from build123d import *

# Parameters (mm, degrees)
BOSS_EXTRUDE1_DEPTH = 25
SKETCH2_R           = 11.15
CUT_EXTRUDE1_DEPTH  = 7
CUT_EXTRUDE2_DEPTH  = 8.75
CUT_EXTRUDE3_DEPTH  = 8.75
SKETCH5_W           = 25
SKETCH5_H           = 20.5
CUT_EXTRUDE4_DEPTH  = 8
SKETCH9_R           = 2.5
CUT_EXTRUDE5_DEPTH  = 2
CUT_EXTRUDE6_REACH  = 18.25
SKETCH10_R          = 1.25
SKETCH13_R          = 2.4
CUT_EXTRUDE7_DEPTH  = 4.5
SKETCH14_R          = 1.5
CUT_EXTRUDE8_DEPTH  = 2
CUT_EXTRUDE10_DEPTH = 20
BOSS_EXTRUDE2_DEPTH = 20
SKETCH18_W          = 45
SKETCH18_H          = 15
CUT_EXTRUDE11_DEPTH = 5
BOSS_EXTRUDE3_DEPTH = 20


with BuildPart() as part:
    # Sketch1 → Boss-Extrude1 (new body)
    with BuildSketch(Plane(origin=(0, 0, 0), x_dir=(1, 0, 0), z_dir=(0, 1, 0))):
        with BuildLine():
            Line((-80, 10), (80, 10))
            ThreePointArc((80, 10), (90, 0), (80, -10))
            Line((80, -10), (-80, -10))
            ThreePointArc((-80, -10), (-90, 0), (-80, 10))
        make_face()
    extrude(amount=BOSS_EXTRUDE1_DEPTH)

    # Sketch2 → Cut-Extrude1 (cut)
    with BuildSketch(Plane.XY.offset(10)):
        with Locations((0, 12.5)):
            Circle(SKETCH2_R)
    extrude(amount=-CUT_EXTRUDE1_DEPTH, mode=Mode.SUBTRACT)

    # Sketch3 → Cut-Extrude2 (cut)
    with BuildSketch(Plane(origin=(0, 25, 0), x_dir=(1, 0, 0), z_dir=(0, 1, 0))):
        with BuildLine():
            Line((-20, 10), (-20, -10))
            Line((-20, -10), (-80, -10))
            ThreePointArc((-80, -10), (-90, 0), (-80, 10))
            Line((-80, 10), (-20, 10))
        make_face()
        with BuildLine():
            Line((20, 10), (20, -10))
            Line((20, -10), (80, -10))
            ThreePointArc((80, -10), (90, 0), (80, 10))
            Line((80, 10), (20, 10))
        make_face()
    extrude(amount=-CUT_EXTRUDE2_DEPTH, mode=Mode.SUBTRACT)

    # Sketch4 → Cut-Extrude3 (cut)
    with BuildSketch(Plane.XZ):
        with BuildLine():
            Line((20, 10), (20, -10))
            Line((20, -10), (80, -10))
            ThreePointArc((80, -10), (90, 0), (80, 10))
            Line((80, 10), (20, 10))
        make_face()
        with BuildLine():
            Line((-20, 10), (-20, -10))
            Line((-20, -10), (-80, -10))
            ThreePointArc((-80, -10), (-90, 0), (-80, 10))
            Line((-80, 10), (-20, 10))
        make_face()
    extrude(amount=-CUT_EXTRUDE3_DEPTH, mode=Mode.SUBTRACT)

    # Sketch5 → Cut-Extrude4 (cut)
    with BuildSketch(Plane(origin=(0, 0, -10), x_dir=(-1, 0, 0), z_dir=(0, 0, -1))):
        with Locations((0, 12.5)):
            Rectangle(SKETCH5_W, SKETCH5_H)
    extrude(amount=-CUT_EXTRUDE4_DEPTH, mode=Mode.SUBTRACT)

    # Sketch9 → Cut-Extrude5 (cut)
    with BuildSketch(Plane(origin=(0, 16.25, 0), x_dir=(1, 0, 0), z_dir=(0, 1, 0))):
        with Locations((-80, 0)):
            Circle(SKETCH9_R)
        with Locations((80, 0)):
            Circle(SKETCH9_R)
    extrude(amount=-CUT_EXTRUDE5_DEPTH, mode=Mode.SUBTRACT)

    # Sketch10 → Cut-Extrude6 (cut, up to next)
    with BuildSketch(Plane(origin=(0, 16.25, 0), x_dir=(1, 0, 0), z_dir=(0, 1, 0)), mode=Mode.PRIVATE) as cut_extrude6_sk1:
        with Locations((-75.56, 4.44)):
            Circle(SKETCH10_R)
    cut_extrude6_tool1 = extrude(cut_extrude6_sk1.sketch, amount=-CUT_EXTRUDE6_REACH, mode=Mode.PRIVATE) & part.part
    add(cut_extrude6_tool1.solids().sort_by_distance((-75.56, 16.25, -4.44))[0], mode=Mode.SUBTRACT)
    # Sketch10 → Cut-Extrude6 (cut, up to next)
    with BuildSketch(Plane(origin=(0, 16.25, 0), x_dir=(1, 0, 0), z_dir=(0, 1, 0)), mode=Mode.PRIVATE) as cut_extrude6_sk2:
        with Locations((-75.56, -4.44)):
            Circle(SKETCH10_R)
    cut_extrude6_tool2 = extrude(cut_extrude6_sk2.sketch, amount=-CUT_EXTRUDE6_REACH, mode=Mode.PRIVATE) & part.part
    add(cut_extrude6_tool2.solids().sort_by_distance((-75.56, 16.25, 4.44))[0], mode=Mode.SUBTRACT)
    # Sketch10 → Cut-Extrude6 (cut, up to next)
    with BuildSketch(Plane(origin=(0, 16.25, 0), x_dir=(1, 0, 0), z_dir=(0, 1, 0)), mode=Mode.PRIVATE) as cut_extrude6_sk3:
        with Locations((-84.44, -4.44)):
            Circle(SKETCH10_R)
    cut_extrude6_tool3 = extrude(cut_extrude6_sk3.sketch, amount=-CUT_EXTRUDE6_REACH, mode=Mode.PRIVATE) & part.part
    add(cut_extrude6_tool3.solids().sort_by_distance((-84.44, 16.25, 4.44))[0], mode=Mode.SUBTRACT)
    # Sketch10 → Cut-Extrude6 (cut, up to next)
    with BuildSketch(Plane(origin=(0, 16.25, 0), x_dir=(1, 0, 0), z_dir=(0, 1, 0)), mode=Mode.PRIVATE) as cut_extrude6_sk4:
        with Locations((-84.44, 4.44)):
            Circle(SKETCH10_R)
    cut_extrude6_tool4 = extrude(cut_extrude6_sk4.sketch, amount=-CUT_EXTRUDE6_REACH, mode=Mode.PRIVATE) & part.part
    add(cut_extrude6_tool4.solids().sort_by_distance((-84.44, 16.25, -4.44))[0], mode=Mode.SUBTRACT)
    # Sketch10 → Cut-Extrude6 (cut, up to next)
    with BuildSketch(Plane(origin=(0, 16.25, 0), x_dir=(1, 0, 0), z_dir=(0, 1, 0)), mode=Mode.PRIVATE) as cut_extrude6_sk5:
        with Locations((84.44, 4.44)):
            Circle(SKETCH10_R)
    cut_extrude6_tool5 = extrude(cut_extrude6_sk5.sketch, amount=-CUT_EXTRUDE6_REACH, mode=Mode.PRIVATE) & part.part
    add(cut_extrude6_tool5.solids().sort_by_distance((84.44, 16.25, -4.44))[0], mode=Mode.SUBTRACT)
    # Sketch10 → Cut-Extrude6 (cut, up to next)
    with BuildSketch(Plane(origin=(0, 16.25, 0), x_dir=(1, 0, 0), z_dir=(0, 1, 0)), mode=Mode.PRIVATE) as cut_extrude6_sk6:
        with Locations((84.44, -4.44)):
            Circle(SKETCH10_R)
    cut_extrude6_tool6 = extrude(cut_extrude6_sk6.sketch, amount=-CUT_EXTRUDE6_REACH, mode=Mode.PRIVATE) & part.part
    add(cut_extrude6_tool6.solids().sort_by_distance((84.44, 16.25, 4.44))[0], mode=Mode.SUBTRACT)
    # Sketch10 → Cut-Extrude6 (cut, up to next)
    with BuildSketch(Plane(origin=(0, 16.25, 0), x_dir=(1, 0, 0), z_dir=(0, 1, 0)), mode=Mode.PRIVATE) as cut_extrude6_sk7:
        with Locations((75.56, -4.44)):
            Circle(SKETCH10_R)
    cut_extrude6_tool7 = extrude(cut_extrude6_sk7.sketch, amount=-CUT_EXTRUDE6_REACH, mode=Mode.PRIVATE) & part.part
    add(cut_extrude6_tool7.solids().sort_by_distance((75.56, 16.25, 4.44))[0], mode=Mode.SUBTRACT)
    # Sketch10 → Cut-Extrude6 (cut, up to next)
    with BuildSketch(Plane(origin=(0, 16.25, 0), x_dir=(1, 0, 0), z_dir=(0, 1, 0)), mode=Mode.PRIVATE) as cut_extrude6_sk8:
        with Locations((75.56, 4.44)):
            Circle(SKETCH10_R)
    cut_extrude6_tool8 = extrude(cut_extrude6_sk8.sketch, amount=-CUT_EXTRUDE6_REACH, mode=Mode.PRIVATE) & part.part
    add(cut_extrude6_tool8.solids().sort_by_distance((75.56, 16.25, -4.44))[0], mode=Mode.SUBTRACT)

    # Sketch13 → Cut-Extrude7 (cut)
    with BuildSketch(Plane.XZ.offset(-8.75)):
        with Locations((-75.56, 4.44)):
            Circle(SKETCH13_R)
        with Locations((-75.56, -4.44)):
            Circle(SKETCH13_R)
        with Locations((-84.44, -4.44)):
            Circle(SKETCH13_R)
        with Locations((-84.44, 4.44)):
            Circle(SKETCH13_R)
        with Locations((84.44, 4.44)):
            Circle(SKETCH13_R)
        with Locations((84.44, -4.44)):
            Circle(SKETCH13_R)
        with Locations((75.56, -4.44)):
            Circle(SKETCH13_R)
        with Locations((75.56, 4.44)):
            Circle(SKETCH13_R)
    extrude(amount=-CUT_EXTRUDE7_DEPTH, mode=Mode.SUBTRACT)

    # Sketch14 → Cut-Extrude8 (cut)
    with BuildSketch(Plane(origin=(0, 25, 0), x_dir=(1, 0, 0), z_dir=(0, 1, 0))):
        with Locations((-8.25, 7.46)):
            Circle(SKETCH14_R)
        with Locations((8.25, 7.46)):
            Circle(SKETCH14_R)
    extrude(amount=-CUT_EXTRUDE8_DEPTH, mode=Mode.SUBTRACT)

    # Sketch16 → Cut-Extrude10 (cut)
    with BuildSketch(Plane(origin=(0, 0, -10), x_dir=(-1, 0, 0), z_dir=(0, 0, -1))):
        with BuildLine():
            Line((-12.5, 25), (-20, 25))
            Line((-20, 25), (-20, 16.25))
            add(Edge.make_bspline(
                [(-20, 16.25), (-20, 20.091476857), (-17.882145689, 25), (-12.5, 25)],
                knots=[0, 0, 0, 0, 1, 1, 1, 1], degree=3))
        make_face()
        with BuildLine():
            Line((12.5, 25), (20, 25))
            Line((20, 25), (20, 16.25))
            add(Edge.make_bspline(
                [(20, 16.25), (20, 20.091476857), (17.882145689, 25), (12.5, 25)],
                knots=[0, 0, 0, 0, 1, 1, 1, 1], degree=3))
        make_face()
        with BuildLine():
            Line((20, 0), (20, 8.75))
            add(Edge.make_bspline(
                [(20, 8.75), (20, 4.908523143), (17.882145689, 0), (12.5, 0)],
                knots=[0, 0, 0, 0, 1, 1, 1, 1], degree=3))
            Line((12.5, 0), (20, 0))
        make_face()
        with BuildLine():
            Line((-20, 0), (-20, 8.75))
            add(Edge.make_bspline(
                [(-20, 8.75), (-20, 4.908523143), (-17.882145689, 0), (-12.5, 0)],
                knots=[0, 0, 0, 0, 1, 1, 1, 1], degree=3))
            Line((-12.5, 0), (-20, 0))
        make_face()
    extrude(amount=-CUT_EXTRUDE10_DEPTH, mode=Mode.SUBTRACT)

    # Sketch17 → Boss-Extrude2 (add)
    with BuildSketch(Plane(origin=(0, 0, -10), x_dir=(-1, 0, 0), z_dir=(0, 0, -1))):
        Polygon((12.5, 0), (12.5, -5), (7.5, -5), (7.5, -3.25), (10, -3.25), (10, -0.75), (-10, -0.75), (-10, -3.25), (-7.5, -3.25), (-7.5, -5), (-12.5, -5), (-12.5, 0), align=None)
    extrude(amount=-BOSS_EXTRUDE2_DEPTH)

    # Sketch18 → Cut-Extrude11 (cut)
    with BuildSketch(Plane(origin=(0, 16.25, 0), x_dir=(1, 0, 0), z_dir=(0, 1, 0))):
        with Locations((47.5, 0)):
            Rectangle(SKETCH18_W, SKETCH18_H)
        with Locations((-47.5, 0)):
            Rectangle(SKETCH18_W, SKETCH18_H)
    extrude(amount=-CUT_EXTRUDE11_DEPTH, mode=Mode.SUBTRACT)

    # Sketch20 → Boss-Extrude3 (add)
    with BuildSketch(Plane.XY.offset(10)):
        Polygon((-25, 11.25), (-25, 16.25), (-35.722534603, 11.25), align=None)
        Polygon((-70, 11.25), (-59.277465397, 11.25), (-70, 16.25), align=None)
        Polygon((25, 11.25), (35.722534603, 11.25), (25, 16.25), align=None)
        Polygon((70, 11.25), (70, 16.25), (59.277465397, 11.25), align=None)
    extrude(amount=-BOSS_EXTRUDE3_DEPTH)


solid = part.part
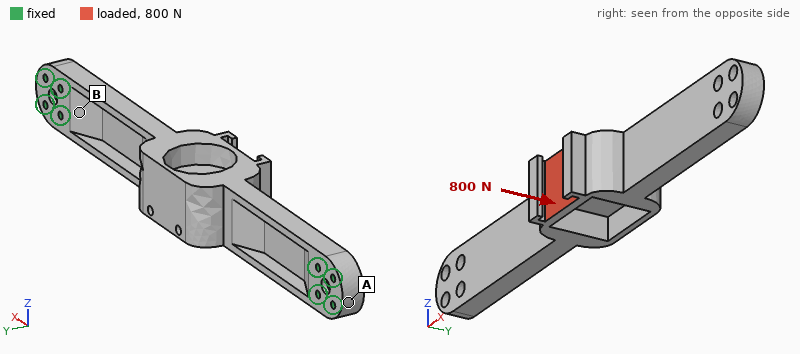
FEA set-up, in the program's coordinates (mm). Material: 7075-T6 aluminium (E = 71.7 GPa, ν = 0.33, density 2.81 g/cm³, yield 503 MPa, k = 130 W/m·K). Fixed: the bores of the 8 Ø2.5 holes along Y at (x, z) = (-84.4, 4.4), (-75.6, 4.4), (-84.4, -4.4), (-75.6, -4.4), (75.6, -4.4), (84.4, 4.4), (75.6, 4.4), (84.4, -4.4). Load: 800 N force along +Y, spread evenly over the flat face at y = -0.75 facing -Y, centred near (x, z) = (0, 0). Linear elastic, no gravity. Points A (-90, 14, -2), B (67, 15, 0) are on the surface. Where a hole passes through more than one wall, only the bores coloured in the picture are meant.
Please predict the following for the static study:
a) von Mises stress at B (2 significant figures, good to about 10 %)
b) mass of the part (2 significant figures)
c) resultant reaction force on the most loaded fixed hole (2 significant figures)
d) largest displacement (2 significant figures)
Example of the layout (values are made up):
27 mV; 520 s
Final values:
37 MPa; 77 g; 740 N; 0.24 mm
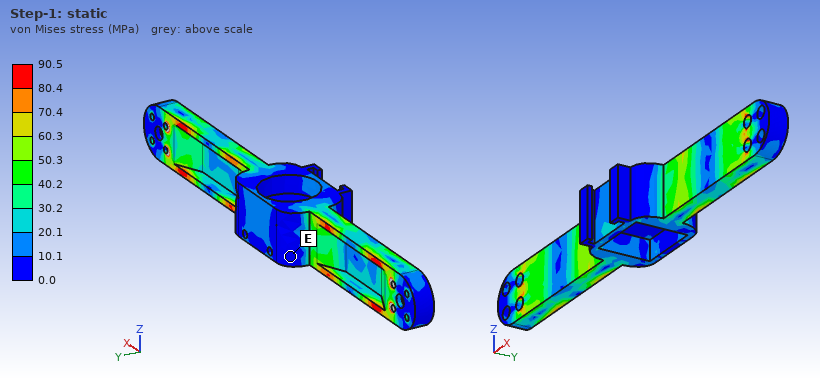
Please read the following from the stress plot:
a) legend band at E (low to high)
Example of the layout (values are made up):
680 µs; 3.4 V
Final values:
0.0 to 10.1 MPa
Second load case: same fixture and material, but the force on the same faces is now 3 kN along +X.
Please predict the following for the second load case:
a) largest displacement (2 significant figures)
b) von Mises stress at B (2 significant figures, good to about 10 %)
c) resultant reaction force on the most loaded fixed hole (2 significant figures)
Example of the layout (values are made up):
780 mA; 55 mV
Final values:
98 µm; 28 MPa; 790 N
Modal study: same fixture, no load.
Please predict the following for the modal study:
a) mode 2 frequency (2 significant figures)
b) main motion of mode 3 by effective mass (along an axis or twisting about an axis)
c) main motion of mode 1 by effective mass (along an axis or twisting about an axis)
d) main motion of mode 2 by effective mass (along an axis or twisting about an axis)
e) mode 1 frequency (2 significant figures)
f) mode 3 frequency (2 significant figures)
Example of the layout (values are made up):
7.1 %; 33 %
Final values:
1600 Hz; along Z; along Y; along Z; 1300 Hz; 2600 Hz
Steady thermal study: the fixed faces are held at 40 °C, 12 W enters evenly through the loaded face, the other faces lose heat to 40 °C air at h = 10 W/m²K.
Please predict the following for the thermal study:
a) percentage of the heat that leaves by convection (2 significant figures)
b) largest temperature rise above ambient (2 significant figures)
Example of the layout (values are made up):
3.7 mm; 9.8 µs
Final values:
19 %; 30 K
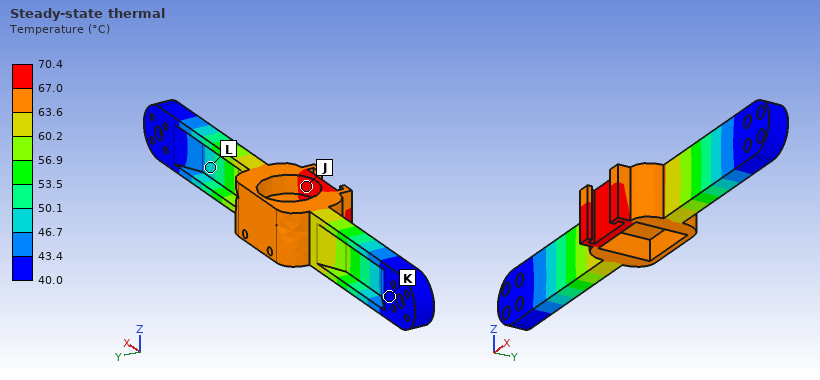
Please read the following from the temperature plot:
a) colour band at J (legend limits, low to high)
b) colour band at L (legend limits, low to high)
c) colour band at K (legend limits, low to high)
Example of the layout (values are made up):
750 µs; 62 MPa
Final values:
67.0 to 70.4 °C; 46.7 to 50.1 °C; 40.0 to 43.4 °C
